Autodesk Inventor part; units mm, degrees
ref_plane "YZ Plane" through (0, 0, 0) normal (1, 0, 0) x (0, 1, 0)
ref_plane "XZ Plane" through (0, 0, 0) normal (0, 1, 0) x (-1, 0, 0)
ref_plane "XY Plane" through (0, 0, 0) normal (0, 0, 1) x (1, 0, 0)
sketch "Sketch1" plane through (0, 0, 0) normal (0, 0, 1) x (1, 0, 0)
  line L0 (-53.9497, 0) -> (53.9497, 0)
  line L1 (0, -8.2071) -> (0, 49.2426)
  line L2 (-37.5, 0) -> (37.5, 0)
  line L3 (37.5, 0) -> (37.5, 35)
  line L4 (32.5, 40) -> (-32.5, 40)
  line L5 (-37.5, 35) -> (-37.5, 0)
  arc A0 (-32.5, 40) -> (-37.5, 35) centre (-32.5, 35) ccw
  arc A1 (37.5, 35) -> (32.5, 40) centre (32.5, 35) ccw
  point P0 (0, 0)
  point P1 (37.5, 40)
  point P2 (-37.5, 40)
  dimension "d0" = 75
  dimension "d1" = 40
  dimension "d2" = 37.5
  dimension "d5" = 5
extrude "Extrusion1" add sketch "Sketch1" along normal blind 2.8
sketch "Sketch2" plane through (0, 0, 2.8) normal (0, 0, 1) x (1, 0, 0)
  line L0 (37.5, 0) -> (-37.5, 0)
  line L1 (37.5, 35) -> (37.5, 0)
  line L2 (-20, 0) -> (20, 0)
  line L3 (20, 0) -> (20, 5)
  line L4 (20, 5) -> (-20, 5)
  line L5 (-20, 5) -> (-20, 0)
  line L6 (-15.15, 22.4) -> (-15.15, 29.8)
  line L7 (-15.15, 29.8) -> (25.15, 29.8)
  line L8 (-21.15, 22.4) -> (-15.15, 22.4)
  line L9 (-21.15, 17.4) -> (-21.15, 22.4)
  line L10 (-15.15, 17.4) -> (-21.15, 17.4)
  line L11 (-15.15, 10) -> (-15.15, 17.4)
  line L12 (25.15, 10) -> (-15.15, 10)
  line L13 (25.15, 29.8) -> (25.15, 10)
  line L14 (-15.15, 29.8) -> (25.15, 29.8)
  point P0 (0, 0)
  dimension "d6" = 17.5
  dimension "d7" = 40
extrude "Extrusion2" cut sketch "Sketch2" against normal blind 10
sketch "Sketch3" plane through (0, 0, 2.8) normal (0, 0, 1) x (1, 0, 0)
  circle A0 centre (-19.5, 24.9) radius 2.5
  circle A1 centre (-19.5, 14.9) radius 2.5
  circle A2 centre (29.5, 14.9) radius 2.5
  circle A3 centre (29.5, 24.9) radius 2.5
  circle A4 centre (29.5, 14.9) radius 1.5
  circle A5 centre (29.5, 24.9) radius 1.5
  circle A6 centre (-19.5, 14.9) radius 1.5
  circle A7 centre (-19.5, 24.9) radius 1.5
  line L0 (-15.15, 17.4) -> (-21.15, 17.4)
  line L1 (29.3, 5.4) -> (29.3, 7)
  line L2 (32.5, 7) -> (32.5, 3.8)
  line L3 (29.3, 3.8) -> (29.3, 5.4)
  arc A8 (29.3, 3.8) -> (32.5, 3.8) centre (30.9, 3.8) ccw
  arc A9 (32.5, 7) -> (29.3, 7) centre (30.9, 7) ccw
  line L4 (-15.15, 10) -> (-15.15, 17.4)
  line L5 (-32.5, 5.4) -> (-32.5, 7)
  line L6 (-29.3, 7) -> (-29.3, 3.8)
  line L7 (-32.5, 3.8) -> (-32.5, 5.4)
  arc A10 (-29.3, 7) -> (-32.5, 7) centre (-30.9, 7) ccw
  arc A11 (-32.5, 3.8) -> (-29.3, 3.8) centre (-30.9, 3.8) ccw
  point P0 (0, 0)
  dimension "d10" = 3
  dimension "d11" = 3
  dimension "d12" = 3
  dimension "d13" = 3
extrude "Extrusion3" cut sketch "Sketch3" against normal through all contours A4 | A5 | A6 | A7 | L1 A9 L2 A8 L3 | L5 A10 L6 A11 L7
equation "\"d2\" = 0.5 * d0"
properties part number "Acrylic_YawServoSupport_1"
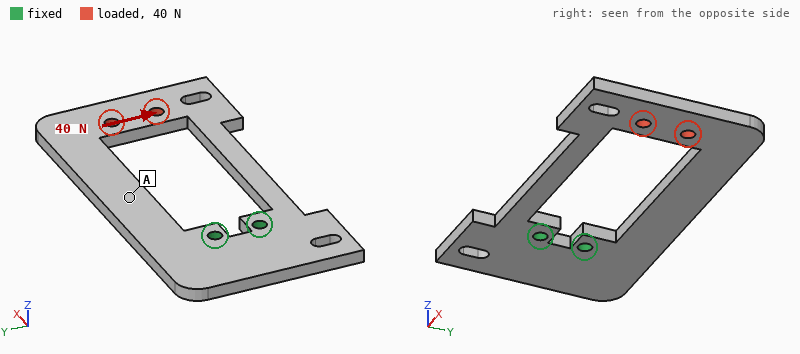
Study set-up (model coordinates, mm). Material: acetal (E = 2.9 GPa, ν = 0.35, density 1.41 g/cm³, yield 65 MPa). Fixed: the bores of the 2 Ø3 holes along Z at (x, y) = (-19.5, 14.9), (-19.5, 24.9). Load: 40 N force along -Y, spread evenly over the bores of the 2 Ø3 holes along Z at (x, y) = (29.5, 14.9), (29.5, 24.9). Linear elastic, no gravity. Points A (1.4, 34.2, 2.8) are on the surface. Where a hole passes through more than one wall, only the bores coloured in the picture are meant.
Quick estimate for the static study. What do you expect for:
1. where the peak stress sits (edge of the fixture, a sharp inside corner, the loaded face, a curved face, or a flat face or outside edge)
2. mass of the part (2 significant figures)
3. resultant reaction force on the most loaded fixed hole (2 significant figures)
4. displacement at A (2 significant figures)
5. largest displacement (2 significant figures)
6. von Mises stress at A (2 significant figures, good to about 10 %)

edge of the fixture
7.5 g
140 N
0.37 mm
1.0 mm
3.0 MPa
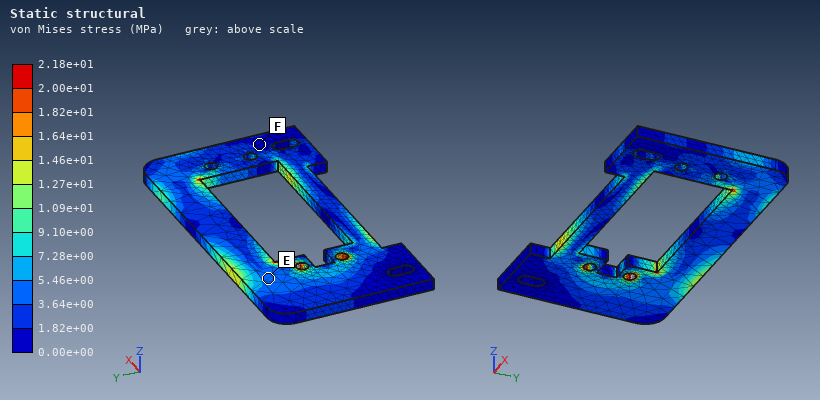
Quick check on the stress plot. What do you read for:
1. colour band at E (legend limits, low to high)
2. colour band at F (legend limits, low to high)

3.64e+00 to 5.46e+00 MPa
0.00e+00 to 1.82e+00 MPa
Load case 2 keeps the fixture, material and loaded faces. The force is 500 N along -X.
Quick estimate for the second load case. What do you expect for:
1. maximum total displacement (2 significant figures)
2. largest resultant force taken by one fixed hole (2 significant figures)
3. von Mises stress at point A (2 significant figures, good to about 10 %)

0.62 mm
280 N
9.5 MPa
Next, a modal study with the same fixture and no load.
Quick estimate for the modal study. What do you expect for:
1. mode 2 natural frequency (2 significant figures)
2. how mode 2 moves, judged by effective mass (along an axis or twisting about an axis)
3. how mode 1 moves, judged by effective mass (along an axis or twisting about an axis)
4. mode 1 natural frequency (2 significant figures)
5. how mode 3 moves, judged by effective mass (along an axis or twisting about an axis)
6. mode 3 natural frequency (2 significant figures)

390 Hz
twisting about X
along Z
130 Hz
along Y
620 Hz
